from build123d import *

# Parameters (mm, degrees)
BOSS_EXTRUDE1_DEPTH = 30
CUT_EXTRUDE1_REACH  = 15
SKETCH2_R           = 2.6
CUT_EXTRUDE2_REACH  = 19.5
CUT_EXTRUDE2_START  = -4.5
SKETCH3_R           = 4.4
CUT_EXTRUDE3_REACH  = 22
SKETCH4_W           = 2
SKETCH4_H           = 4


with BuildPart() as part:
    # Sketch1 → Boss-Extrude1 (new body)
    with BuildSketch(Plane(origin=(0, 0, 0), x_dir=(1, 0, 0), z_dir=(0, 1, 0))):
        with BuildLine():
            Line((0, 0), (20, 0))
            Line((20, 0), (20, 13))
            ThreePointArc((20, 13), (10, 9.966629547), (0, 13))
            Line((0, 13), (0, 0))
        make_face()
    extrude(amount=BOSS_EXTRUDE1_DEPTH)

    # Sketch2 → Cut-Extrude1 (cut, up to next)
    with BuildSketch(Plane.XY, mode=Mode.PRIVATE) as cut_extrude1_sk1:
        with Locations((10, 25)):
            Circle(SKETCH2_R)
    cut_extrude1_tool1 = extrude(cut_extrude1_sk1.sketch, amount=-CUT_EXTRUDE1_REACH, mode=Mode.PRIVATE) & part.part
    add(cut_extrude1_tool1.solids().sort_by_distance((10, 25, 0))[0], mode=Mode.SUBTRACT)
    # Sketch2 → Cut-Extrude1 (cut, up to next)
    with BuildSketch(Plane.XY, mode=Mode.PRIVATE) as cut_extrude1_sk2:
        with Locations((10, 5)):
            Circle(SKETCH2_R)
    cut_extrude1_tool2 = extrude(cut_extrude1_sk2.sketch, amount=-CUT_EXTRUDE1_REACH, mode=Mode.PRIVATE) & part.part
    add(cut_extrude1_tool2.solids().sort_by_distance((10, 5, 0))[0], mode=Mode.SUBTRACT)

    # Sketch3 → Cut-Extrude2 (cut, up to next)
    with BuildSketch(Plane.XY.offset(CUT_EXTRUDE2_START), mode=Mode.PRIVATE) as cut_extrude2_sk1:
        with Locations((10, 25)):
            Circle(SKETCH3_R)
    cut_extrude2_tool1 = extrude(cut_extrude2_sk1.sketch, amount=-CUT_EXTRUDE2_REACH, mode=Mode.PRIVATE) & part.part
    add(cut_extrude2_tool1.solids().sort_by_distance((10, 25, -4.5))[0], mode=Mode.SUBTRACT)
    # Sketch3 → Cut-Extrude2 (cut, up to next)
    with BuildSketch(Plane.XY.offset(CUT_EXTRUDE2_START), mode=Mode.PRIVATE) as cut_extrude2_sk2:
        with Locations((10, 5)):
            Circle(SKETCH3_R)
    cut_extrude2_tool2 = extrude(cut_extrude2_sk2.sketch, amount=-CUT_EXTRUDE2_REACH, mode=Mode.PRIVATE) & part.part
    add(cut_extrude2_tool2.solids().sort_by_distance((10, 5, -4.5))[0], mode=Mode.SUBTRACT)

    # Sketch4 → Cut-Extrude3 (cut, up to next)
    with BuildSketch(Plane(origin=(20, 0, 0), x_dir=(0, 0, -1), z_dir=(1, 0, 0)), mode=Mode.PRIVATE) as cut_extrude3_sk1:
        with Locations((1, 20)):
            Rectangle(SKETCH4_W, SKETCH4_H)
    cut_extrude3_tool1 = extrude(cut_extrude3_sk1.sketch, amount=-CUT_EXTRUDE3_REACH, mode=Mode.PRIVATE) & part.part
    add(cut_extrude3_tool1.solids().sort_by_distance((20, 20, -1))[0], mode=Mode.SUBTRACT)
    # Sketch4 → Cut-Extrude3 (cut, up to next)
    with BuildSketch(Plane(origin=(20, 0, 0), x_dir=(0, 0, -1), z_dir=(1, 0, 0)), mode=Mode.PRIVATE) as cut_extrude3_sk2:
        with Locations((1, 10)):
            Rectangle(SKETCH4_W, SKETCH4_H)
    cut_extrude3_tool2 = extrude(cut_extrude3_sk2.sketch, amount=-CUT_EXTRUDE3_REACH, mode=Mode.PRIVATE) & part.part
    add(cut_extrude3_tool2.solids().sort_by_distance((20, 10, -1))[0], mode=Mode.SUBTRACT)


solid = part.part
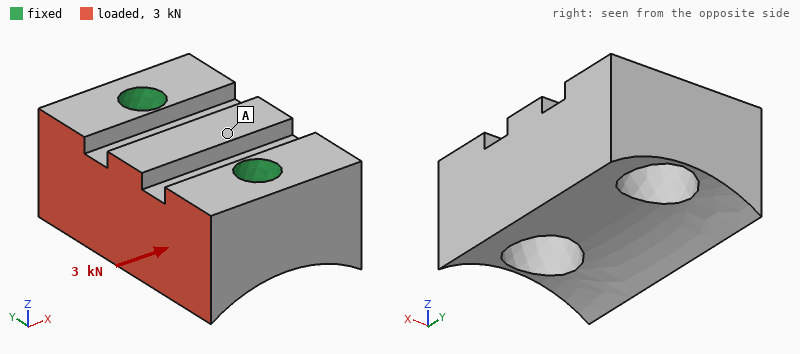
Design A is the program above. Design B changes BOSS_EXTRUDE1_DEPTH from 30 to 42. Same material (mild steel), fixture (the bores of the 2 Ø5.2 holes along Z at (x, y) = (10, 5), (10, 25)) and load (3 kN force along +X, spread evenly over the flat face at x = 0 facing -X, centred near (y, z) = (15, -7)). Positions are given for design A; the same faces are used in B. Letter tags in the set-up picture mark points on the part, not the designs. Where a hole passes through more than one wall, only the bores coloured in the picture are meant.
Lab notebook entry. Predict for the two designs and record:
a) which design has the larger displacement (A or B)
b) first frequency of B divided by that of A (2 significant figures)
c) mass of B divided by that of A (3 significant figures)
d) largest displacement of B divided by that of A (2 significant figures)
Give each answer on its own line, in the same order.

B
0.78
1.49
1.1
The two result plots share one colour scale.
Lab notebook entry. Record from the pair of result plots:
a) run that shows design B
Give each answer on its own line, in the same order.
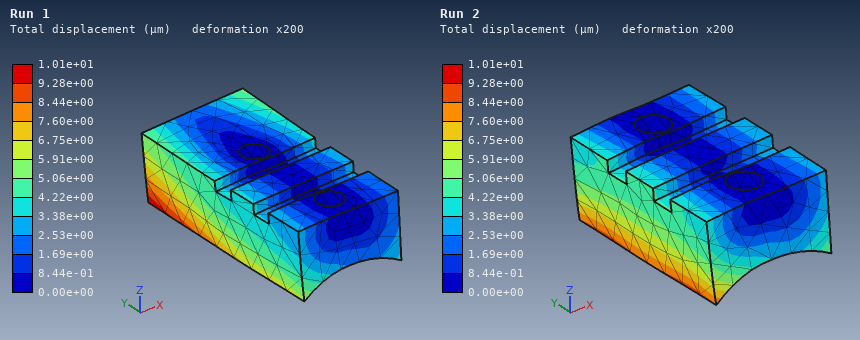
Run 1
